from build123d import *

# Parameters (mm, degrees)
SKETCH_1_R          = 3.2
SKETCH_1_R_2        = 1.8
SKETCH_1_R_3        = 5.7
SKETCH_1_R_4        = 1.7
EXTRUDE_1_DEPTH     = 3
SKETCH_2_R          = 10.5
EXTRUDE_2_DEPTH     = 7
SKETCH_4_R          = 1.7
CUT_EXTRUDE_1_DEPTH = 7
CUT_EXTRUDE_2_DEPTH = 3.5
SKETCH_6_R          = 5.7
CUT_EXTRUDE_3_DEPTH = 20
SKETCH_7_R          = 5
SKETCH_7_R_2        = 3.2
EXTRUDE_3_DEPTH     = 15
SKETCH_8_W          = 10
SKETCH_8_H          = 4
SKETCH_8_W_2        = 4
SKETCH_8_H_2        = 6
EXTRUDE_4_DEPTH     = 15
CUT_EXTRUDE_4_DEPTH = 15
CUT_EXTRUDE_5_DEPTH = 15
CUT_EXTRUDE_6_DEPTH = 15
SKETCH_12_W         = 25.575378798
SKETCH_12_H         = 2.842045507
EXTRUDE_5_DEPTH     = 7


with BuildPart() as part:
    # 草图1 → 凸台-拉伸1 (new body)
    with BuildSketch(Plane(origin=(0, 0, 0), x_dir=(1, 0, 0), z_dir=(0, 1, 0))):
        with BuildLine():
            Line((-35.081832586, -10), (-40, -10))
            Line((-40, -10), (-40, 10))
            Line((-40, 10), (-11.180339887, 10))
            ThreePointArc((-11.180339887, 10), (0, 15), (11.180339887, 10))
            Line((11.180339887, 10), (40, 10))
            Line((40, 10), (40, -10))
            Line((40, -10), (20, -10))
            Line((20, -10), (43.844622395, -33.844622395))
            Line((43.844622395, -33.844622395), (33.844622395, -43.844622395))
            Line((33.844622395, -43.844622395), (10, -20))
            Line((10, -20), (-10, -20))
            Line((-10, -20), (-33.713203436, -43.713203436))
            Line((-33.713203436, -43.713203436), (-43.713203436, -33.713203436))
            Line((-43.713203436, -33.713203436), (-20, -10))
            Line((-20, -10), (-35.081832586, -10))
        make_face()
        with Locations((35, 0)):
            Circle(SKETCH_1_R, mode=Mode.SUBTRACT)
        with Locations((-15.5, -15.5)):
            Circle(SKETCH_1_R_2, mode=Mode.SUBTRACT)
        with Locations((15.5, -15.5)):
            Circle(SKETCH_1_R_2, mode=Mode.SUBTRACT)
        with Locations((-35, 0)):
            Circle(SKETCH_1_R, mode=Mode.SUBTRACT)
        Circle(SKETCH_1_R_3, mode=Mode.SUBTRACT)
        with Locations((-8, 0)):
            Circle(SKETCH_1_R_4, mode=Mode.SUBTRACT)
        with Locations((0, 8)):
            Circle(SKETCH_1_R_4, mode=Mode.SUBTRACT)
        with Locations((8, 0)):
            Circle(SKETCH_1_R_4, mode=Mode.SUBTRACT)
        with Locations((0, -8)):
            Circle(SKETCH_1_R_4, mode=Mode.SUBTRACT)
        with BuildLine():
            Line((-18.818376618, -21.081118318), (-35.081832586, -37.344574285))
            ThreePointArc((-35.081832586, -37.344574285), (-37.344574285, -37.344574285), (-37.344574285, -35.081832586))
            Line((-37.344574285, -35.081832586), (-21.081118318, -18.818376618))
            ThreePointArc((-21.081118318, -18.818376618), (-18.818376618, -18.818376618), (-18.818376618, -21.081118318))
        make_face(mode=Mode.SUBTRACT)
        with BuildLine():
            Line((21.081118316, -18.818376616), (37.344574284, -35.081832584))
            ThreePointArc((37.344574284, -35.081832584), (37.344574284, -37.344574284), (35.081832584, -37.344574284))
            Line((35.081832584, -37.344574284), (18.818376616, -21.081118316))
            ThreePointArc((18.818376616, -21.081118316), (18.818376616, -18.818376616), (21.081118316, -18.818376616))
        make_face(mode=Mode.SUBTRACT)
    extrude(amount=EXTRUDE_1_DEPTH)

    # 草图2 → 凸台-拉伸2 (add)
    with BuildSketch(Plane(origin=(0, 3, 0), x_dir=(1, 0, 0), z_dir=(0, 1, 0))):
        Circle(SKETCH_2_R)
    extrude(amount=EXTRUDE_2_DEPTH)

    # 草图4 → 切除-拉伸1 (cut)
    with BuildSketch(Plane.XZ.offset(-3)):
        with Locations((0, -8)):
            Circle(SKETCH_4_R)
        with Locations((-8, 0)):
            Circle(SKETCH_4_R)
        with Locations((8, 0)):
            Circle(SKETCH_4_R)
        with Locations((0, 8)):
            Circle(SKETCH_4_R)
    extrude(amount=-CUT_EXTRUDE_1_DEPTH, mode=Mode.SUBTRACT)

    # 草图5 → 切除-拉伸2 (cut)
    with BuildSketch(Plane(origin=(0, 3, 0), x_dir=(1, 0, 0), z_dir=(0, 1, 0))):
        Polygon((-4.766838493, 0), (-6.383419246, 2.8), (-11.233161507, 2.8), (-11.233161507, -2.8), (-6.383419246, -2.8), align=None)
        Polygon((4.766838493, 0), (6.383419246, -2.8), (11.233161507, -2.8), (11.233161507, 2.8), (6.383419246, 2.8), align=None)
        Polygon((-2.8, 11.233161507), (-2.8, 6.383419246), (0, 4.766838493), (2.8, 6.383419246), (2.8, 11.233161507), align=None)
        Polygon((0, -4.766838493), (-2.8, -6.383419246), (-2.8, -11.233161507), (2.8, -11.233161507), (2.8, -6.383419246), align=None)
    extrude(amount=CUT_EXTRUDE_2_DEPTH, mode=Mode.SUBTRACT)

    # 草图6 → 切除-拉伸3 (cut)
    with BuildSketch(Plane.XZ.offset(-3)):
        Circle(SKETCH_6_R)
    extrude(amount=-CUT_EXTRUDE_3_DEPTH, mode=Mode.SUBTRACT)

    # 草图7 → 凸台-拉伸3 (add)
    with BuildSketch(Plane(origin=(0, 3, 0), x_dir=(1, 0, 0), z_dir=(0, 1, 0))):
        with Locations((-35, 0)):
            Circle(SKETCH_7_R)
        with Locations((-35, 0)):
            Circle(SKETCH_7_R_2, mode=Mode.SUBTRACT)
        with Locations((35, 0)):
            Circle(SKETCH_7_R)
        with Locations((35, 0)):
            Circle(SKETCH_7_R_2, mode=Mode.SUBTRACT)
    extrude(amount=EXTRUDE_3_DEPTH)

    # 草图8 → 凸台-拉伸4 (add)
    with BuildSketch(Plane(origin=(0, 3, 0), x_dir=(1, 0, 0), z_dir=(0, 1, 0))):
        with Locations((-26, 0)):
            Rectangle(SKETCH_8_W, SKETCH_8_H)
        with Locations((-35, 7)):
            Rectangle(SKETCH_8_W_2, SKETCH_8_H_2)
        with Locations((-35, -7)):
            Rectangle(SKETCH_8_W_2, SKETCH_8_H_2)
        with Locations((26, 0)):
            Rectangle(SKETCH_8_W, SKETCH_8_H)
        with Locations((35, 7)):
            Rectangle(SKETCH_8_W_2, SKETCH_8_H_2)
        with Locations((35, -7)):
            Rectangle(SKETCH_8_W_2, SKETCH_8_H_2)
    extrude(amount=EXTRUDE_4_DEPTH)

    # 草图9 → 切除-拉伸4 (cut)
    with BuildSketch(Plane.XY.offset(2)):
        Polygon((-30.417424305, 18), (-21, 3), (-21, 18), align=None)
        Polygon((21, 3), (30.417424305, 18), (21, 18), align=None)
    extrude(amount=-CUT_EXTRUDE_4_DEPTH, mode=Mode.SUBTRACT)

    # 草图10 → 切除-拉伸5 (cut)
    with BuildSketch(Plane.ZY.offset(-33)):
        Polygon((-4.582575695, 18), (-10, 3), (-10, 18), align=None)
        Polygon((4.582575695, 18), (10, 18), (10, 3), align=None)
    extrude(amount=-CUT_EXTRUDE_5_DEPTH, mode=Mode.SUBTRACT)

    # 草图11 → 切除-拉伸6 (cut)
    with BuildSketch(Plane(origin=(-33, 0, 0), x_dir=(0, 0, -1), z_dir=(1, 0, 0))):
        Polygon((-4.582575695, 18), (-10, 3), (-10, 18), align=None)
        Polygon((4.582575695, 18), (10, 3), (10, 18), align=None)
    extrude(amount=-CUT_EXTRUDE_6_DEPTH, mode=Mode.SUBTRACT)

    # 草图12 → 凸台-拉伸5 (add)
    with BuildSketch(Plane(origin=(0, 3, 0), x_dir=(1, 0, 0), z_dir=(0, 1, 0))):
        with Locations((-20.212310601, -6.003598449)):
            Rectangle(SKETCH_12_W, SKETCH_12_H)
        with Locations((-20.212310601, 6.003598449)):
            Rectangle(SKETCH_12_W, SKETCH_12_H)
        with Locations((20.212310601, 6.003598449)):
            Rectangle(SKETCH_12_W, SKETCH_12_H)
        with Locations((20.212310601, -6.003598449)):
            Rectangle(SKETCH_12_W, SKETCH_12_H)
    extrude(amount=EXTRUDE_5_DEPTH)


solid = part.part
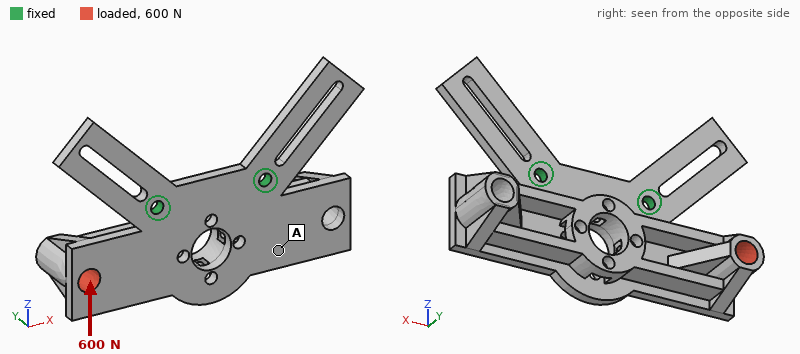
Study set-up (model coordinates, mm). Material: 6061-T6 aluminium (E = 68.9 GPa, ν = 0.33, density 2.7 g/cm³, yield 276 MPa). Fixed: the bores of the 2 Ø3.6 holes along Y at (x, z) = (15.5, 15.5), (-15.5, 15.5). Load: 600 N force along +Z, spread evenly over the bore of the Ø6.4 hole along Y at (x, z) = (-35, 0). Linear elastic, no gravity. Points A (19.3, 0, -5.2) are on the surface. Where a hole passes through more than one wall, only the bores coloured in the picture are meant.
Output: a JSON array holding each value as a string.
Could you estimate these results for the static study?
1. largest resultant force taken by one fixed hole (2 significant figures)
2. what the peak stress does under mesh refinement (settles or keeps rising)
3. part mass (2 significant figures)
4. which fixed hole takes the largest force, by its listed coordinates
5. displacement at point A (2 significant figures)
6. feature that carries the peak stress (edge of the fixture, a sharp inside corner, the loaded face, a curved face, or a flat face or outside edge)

["960 N", "keeps rising", "36 g", "(-15.5, 15.5)", "0.082 mm", "edge of the fixture"]
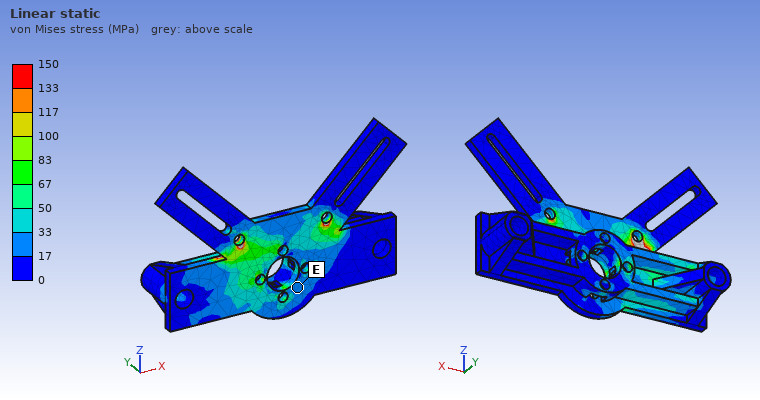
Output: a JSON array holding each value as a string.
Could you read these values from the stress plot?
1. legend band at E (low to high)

["17 to 33 MPa"]
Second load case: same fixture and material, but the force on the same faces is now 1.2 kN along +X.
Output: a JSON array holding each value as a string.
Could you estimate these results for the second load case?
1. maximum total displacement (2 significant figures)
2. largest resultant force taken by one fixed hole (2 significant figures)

["0.17 mm", "850 N"]
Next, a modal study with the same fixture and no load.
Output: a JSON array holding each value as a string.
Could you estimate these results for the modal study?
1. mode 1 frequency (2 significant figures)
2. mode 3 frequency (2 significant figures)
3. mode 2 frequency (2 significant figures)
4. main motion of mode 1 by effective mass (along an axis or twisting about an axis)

["1700 Hz", "2300 Hz", "2300 Hz", "along Y"]
